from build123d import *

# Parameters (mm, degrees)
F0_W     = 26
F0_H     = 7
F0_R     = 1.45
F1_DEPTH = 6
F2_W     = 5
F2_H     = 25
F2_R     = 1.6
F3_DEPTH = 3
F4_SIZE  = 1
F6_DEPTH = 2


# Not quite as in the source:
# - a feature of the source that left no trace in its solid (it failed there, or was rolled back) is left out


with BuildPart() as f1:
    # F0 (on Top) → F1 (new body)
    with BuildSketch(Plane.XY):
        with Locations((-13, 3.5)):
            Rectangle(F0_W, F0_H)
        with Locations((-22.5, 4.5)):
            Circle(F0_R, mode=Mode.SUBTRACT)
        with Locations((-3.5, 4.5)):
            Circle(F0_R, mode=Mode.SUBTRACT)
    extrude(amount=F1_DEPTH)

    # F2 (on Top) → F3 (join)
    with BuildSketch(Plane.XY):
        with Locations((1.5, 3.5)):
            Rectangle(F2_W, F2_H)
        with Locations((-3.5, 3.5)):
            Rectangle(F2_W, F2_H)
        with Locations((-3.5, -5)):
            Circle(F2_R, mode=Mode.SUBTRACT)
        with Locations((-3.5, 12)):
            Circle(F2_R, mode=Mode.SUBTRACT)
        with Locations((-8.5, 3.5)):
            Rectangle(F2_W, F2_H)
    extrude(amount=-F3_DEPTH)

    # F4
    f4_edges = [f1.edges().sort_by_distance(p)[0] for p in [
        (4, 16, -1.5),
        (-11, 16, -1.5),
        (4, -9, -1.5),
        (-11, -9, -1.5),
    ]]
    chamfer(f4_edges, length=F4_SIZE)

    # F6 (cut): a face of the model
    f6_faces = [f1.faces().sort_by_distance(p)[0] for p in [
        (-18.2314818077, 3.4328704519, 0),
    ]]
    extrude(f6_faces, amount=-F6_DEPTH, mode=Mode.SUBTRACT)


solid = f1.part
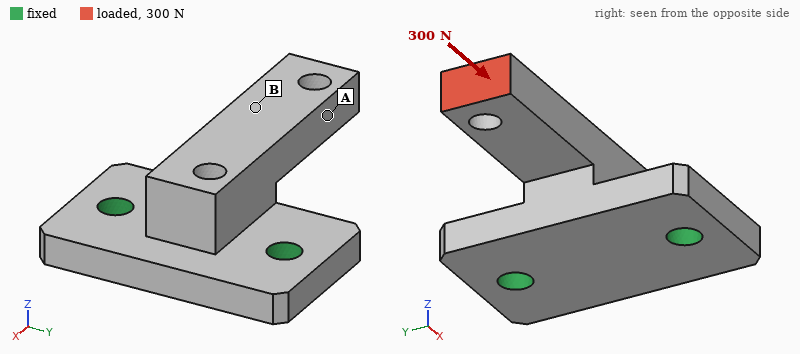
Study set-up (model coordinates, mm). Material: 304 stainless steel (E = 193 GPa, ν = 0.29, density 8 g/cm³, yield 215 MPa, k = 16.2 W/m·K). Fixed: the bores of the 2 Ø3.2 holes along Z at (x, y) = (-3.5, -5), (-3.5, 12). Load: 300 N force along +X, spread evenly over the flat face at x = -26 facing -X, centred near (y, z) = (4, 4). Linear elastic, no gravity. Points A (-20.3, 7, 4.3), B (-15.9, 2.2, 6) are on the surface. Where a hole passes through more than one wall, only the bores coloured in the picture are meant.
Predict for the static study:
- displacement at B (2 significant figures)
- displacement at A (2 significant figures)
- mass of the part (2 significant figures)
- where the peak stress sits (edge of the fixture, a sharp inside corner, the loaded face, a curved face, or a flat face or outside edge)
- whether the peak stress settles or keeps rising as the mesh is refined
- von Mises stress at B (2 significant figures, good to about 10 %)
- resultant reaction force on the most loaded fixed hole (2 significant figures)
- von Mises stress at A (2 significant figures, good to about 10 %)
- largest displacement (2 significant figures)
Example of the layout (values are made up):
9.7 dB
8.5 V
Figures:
7.7 µm
9.5 µm
15 g
edge of the fixture
keeps rising
10 MPa
150 N
23 MPa
13 µm
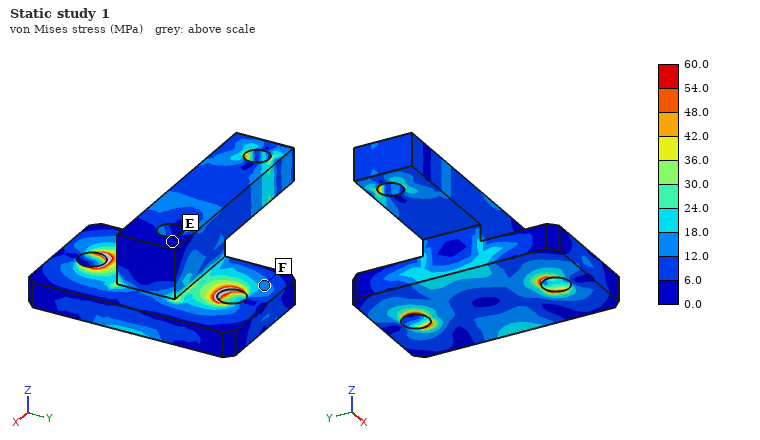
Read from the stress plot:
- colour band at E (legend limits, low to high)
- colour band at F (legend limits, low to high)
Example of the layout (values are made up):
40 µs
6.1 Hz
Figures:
0.0 to 6.0 MPa
12.0 to 18.0 MPa
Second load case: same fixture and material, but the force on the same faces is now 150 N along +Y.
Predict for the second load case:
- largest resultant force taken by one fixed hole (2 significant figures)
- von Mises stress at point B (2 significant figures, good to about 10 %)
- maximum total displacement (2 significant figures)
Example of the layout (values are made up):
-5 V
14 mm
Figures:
220 N
19 MPa
22 µm
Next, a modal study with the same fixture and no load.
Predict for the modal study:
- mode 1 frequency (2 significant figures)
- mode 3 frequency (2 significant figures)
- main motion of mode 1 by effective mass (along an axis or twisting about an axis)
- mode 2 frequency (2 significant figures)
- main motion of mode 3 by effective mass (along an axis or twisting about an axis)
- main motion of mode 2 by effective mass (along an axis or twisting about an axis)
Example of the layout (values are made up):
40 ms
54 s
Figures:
7400 Hz
22 kHz
along Z
13 kHz
along X
along Y
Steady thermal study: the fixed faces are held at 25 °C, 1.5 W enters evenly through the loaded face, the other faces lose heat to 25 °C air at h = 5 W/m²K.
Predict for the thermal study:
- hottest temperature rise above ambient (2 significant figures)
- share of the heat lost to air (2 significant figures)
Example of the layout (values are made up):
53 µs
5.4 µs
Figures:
77 K
7.5 %
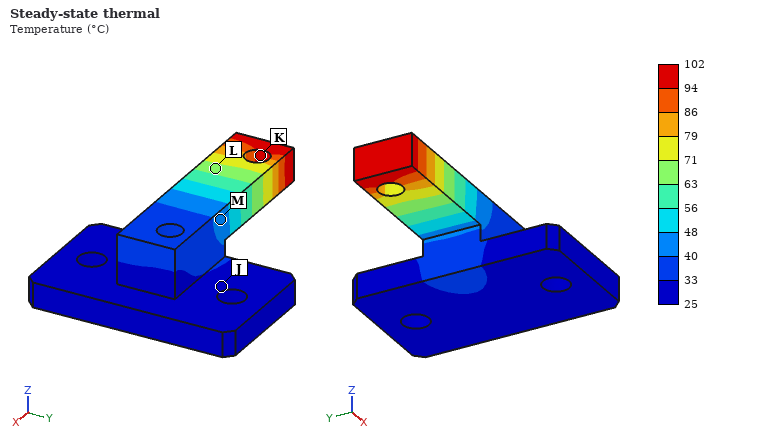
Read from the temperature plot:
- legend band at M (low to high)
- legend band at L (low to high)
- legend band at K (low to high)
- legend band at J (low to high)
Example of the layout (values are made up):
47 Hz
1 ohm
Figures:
40 to 48 °C
63 to 71 °C
94 to 102 °C
25 to 33 °C
